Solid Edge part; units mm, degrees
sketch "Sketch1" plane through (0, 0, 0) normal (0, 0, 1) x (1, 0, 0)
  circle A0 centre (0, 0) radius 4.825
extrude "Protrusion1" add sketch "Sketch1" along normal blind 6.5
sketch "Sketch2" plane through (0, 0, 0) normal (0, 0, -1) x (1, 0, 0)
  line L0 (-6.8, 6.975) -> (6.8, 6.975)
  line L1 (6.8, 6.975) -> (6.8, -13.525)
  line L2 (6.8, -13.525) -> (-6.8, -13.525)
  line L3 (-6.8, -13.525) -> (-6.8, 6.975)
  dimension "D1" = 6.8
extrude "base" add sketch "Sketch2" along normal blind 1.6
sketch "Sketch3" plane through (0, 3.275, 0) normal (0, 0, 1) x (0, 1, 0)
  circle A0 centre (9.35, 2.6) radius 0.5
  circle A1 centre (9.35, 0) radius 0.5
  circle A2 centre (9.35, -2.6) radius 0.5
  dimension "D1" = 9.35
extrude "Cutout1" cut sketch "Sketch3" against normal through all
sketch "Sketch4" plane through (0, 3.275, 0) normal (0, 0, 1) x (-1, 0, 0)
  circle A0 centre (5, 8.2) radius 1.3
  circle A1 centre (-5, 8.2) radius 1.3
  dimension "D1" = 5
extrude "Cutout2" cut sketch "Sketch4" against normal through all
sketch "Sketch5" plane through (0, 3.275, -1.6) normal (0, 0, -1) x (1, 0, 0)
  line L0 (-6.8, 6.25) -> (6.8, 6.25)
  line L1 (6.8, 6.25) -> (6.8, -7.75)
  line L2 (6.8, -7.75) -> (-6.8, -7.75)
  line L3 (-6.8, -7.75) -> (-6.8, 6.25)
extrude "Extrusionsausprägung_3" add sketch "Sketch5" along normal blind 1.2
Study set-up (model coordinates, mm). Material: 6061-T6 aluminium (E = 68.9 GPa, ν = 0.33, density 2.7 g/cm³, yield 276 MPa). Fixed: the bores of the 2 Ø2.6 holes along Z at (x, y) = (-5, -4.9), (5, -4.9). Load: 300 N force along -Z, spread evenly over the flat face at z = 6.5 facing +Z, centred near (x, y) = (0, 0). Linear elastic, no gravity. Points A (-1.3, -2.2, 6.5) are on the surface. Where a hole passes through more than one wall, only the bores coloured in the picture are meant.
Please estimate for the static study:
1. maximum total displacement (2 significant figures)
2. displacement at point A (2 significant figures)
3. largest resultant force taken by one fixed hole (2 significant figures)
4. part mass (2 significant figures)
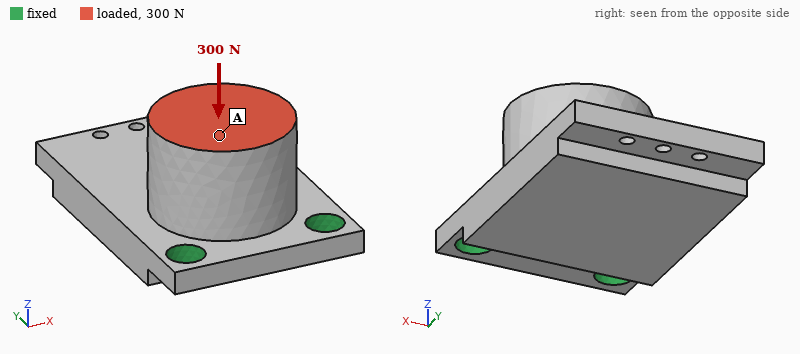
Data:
84 µm
35 µm
150 N
3.0 g
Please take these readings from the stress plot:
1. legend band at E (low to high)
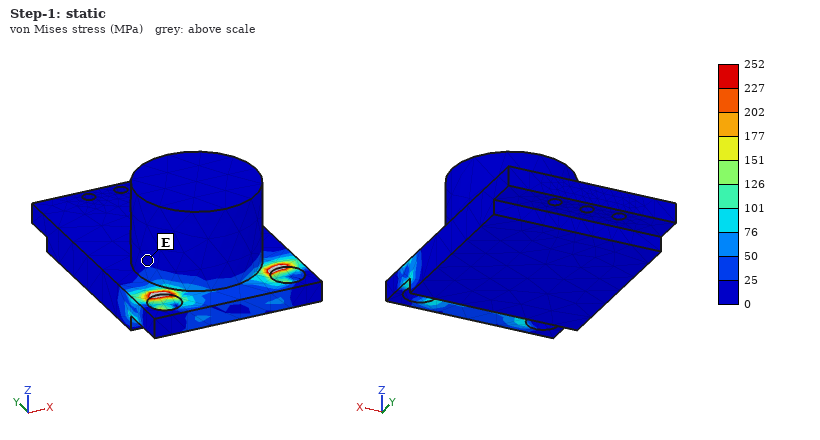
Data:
0 to 25 MPa
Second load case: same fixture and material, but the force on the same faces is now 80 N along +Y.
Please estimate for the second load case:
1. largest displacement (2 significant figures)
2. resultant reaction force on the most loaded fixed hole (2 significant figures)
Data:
43 µm
44 N
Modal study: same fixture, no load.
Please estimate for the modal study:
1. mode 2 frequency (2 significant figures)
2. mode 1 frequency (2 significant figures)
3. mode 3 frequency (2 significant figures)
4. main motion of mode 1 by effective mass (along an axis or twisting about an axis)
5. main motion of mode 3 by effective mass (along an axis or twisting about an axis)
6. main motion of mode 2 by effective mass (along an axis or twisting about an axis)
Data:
24 kHz
5400 Hz
26 kHz
along Z
along X
along X
